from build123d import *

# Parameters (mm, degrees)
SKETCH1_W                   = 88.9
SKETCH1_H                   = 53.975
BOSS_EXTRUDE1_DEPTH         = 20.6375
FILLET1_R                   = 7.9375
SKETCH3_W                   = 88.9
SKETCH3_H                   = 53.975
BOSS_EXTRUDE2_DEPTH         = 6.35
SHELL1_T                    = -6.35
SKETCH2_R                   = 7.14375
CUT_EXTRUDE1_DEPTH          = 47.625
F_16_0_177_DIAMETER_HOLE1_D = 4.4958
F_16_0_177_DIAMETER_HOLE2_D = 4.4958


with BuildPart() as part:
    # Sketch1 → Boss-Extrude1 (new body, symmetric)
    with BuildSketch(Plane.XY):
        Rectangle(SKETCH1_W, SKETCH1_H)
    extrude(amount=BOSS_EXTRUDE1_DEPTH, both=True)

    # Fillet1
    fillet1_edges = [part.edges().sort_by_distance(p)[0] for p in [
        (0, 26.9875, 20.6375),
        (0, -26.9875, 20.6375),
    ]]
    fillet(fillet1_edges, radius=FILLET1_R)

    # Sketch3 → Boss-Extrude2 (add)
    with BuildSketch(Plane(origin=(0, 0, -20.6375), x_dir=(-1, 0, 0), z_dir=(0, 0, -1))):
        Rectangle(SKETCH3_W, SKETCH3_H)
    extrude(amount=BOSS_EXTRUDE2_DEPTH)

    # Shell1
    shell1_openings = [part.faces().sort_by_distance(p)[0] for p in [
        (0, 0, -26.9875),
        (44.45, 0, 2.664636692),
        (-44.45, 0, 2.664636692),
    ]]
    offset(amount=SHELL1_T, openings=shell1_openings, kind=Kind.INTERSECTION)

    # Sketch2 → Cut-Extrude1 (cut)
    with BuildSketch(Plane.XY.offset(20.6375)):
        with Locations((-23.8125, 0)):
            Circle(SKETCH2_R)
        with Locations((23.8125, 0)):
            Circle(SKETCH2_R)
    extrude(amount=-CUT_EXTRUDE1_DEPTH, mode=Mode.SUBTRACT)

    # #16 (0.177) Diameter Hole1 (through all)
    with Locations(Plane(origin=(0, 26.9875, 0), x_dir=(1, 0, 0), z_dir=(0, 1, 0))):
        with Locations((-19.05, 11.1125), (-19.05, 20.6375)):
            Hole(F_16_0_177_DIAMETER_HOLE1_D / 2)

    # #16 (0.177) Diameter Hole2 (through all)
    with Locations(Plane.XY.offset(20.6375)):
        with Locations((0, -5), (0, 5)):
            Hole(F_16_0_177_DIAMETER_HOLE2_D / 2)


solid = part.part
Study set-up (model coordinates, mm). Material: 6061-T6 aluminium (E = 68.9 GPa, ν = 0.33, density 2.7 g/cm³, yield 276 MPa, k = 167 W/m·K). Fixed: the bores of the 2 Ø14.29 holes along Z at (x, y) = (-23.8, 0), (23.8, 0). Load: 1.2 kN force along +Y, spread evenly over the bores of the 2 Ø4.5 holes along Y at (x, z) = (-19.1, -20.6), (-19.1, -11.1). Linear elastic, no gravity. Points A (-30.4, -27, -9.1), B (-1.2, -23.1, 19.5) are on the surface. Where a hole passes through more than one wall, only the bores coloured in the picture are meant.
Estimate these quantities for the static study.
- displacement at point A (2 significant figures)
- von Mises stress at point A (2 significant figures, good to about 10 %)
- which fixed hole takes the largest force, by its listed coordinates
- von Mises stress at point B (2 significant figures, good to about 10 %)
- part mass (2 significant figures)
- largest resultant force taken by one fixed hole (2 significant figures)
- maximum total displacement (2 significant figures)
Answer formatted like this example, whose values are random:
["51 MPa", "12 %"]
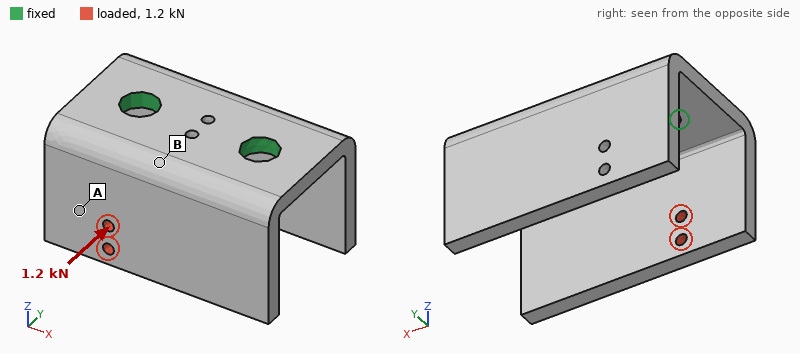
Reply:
["0.29 mm", "17 MPa", "(-23.8, 0)", "43 MPa", "190 g", "1.0 kN", "0.50 mm"]
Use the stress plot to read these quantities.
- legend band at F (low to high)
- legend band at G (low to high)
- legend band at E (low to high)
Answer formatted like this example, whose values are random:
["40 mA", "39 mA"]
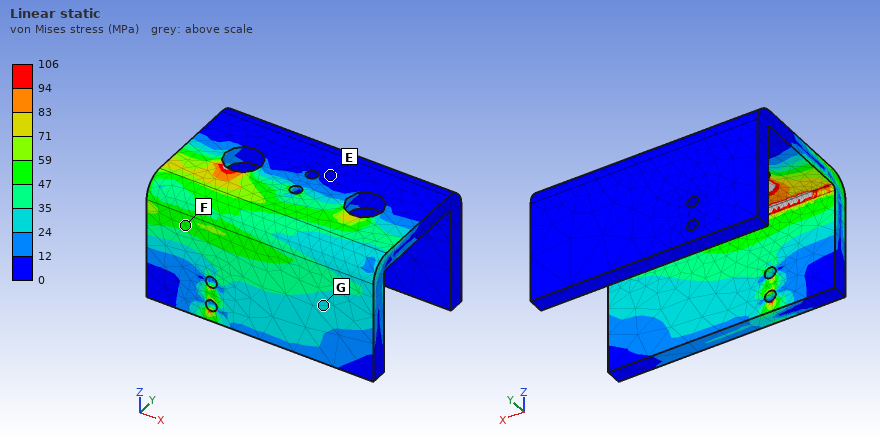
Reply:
["47 to 59 MPa", "24 to 35 MPa", "0 to 12 MPa"]
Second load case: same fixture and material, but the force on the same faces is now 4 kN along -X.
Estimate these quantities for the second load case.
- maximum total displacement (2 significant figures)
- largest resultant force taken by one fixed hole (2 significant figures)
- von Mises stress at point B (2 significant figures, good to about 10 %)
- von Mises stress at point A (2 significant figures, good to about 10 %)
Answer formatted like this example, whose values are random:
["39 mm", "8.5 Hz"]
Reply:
["0.22 mm", "3.4 kN", "24 MPa", "7.5 MPa"]
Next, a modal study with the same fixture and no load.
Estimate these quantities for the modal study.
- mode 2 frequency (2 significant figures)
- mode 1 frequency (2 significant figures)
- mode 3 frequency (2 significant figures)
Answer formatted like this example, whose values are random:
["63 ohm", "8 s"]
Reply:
["1600 Hz", "1600 Hz", "2800 Hz"]
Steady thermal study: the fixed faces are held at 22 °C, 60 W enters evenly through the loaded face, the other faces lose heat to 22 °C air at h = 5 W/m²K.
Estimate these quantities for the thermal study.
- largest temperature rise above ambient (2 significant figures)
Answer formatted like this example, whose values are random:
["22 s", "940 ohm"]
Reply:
["54 K"]
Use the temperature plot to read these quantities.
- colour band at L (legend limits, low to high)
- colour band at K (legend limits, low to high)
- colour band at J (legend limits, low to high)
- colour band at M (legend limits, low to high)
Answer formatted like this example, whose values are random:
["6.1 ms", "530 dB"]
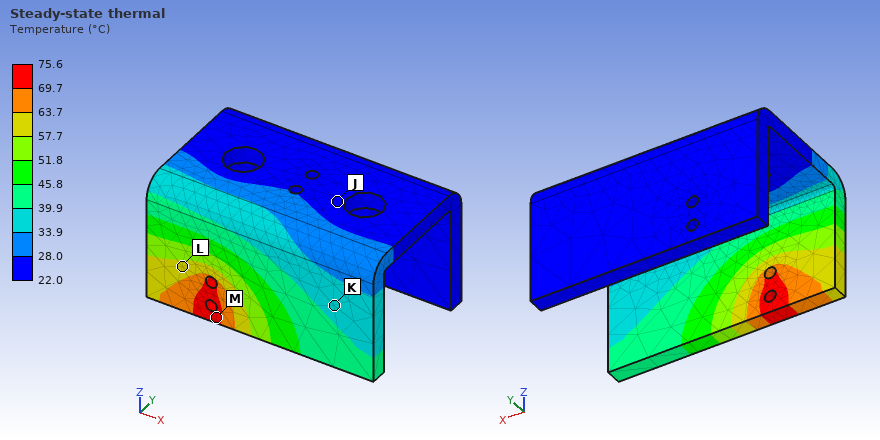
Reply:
["57.7 to 63.7 °C", "33.9 to 39.9 °C", "22.0 to 28.0 °C", "69.7 to 75.6 °C"]
